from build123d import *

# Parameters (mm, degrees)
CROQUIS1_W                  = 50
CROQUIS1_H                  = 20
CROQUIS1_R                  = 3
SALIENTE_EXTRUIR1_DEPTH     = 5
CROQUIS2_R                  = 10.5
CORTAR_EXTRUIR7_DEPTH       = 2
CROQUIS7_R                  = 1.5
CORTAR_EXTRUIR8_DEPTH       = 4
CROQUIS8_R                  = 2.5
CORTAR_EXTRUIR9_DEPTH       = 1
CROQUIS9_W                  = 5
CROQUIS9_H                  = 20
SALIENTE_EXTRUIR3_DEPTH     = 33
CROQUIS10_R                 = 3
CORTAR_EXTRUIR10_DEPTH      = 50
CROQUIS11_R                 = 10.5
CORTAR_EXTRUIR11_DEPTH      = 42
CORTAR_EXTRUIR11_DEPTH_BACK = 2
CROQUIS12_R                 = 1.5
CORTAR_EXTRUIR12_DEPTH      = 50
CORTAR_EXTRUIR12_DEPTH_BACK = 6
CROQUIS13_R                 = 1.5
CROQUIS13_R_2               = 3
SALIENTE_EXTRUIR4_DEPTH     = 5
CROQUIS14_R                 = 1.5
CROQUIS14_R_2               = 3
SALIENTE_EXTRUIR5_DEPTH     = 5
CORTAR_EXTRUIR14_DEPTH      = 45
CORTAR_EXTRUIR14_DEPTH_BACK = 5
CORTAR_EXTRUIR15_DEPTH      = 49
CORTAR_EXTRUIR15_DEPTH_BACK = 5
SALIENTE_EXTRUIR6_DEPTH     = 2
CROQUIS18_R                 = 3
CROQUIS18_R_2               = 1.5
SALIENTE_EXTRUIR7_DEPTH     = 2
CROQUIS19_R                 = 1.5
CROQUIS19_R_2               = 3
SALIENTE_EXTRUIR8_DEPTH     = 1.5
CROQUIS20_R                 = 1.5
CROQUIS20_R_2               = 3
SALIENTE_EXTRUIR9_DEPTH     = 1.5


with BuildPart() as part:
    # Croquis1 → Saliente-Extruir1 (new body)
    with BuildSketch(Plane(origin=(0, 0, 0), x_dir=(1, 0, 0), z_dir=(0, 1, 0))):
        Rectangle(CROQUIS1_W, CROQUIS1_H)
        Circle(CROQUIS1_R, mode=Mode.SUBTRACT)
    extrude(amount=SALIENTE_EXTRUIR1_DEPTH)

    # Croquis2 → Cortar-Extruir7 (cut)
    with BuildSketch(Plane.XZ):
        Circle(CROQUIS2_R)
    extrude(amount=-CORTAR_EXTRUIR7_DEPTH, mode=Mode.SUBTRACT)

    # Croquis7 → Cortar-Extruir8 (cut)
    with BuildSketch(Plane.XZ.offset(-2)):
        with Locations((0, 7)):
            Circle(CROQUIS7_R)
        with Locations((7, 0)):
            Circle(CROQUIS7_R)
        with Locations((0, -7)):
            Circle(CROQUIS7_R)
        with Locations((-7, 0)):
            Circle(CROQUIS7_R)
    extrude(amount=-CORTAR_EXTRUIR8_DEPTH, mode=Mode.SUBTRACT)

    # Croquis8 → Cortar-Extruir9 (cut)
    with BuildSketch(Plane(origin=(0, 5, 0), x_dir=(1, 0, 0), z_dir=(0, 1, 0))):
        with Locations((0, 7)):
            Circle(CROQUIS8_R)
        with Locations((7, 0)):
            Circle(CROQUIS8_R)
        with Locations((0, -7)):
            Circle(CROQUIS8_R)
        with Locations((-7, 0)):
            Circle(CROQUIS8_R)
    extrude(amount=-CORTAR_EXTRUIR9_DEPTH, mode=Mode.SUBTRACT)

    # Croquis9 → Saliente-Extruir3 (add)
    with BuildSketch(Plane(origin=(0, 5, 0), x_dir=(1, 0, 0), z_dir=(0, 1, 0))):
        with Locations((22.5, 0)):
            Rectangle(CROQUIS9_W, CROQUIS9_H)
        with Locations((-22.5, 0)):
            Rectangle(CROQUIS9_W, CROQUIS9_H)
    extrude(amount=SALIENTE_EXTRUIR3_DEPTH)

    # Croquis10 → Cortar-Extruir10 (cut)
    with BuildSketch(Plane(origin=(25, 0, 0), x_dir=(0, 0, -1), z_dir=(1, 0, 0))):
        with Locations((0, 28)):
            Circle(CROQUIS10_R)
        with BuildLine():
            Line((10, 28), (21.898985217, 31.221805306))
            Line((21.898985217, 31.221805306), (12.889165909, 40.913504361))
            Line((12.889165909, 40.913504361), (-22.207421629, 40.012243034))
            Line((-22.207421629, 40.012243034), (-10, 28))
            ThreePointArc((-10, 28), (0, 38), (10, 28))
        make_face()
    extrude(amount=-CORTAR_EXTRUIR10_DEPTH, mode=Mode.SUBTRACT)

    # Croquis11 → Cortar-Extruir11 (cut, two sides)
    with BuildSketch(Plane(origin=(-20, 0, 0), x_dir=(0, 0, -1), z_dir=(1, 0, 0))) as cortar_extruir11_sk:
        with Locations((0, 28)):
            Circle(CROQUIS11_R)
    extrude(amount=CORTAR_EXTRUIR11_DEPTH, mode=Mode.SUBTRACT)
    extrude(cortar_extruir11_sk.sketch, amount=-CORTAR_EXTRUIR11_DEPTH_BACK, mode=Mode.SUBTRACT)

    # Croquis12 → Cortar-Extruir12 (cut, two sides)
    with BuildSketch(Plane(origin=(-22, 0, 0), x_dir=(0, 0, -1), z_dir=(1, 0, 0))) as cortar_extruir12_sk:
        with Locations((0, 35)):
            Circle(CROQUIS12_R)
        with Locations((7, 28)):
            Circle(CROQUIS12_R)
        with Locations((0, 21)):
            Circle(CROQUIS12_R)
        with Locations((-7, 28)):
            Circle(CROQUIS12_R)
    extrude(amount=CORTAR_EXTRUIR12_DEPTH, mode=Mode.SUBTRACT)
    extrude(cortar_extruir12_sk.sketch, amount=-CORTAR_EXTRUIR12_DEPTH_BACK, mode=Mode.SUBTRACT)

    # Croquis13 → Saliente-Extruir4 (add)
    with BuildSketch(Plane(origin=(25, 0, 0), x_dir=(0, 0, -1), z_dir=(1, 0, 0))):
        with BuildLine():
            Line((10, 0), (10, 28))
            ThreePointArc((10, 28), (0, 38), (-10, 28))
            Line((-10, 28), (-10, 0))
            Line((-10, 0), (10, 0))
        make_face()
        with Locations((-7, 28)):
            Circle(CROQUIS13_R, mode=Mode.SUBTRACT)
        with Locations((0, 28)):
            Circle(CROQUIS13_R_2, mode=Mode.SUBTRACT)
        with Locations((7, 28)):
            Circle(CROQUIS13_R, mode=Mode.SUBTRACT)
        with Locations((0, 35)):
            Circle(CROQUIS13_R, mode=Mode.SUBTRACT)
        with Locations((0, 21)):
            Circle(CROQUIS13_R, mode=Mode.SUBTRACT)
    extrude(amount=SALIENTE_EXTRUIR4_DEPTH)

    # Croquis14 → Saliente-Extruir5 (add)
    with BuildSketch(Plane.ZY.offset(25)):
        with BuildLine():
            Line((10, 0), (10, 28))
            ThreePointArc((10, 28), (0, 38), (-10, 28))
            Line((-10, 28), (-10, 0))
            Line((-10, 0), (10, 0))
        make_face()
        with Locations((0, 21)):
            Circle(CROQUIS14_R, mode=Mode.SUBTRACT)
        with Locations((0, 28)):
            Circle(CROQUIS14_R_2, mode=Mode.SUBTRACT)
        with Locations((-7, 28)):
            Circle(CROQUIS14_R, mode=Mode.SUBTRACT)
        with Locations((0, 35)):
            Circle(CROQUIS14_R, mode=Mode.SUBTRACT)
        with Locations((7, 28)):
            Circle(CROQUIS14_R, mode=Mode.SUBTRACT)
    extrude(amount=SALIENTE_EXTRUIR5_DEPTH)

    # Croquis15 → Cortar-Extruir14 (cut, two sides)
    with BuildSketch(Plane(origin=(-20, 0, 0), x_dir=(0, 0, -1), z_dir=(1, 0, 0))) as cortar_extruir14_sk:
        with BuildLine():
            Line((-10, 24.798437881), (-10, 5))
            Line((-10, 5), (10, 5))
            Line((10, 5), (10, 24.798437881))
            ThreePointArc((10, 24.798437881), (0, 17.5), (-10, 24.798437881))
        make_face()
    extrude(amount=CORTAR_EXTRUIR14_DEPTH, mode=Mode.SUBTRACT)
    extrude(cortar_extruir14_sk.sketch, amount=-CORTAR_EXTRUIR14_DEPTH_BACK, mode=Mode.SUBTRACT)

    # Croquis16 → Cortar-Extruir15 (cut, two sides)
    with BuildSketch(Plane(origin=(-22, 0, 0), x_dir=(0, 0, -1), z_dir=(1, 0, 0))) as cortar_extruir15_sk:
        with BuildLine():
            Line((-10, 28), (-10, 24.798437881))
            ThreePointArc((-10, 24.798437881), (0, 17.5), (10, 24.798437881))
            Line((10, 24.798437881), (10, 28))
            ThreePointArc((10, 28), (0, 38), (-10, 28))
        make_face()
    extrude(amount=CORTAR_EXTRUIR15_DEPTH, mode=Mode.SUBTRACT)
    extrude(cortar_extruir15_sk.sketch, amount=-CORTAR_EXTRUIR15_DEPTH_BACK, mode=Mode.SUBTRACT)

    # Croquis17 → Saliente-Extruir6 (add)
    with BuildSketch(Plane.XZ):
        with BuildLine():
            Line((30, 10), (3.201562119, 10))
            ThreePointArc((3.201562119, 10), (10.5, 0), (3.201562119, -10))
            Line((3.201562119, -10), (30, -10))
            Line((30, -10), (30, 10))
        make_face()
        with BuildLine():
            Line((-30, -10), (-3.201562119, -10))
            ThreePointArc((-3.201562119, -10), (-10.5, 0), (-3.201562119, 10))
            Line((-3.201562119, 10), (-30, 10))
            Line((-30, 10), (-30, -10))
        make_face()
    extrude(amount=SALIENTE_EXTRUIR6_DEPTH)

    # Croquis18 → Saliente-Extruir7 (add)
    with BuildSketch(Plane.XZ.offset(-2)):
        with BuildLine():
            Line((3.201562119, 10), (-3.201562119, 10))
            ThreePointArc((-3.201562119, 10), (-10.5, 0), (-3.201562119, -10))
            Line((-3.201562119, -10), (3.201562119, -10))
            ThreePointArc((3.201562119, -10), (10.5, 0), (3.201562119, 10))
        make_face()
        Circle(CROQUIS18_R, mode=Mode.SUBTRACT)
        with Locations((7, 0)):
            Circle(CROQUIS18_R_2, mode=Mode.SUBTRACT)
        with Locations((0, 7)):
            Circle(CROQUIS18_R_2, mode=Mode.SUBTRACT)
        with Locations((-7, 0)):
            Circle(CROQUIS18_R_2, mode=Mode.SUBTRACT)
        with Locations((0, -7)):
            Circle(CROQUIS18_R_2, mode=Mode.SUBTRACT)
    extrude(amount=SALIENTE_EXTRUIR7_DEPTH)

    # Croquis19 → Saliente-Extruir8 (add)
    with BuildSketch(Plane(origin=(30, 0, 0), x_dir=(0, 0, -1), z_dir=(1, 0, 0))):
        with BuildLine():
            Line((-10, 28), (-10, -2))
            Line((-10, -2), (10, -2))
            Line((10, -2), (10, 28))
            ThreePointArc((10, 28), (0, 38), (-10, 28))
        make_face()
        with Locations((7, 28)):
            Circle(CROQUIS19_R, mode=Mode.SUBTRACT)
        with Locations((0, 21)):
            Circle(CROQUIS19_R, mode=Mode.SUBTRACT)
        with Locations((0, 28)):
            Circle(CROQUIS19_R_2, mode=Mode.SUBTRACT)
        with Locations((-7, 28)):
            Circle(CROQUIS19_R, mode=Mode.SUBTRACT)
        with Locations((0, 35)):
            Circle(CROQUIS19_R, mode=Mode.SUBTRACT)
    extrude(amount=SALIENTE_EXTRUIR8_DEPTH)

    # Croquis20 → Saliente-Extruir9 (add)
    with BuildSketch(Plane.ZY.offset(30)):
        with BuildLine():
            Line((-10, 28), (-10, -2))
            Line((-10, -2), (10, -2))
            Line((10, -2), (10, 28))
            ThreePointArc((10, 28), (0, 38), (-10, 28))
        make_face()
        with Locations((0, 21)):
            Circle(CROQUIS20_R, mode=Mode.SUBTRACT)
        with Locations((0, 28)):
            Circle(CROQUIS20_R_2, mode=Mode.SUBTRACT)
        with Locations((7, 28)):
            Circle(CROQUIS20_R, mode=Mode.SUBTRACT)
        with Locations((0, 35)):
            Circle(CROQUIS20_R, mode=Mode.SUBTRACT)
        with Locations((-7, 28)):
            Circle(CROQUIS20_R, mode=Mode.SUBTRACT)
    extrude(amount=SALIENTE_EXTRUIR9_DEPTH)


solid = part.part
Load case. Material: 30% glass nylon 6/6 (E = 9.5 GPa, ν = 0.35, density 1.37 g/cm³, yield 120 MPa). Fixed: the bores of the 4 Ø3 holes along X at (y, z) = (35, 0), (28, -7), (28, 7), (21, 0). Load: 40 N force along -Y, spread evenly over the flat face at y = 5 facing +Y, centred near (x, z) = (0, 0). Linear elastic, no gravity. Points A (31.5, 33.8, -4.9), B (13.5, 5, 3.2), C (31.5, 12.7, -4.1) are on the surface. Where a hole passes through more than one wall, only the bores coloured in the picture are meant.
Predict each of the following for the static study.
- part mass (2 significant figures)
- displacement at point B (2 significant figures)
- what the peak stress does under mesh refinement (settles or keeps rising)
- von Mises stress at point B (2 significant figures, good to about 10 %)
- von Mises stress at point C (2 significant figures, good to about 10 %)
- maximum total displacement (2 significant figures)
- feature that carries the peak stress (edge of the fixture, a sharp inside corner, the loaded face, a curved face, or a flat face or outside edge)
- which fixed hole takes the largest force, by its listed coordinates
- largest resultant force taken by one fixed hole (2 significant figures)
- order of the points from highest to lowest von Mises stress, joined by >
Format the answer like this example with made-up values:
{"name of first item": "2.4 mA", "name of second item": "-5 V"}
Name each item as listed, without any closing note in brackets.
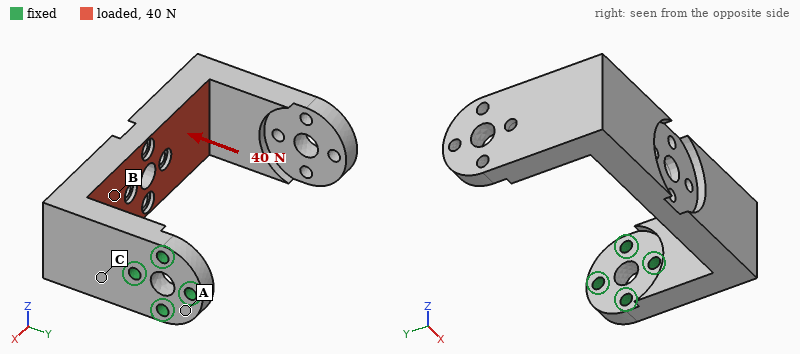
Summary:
{"part mass": "19 g", "displacement at point B": "0.13 mm", "what the peak stress does under mesh refinement": "keeps rising", "von Mises stress at point B": "3.8 MPa", "von Mises stress at point C": "7.5 MPa", "maximum total displacement": "0.77 mm", "feature that carries the peak stress": "edge of the fixture", "which fixed hole takes the largest force, by its listed coordinates": "(21, 0)", "largest resultant force taken by one fixed hole": "84 N", "order of the points from highest to lowest von Mises stress, joined by >": "C > B > A"}
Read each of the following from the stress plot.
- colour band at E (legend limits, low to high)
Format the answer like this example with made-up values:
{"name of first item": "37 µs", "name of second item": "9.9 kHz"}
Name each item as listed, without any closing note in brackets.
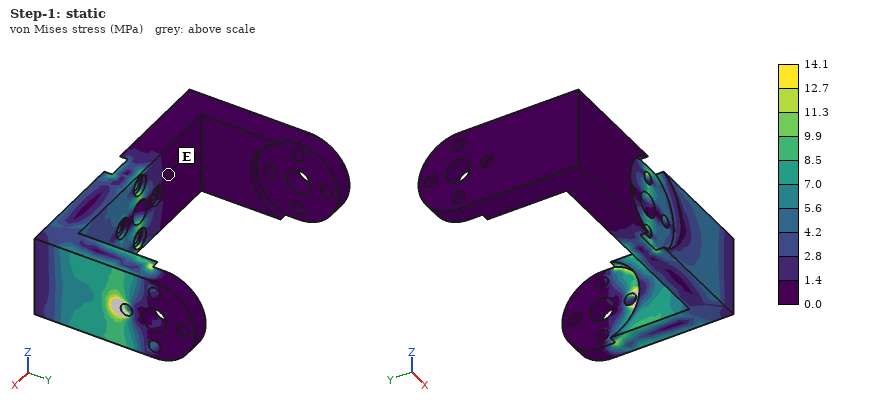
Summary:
{"colour band at E": "0.0 to 1.4 MPa"}
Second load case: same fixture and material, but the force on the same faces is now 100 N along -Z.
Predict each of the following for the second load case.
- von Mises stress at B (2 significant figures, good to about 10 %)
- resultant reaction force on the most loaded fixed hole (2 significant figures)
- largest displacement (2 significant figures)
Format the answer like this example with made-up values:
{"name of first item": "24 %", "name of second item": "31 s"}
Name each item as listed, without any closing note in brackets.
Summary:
{"von Mises stress at B": "3.7 MPa", "resultant reaction force on the most loaded fixed hole": "120 N", "largest displacement": "0.92 mm"}
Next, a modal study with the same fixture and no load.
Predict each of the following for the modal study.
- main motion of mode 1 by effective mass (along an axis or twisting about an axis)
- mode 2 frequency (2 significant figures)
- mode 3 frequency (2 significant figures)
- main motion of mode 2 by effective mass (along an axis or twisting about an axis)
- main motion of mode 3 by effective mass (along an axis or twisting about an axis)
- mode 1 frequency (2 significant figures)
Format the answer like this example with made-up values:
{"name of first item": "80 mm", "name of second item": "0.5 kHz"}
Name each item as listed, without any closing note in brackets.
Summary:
{"main motion of mode 1 by effective mass": "along Y", "mode 2 frequency": "420 Hz", "mode 3 frequency": "1000 Hz", "main motion of mode 2 by effective mass": "along Z", "main motion of mode 3 by effective mass": "along X", "mode 1 frequency": "280 Hz"}
